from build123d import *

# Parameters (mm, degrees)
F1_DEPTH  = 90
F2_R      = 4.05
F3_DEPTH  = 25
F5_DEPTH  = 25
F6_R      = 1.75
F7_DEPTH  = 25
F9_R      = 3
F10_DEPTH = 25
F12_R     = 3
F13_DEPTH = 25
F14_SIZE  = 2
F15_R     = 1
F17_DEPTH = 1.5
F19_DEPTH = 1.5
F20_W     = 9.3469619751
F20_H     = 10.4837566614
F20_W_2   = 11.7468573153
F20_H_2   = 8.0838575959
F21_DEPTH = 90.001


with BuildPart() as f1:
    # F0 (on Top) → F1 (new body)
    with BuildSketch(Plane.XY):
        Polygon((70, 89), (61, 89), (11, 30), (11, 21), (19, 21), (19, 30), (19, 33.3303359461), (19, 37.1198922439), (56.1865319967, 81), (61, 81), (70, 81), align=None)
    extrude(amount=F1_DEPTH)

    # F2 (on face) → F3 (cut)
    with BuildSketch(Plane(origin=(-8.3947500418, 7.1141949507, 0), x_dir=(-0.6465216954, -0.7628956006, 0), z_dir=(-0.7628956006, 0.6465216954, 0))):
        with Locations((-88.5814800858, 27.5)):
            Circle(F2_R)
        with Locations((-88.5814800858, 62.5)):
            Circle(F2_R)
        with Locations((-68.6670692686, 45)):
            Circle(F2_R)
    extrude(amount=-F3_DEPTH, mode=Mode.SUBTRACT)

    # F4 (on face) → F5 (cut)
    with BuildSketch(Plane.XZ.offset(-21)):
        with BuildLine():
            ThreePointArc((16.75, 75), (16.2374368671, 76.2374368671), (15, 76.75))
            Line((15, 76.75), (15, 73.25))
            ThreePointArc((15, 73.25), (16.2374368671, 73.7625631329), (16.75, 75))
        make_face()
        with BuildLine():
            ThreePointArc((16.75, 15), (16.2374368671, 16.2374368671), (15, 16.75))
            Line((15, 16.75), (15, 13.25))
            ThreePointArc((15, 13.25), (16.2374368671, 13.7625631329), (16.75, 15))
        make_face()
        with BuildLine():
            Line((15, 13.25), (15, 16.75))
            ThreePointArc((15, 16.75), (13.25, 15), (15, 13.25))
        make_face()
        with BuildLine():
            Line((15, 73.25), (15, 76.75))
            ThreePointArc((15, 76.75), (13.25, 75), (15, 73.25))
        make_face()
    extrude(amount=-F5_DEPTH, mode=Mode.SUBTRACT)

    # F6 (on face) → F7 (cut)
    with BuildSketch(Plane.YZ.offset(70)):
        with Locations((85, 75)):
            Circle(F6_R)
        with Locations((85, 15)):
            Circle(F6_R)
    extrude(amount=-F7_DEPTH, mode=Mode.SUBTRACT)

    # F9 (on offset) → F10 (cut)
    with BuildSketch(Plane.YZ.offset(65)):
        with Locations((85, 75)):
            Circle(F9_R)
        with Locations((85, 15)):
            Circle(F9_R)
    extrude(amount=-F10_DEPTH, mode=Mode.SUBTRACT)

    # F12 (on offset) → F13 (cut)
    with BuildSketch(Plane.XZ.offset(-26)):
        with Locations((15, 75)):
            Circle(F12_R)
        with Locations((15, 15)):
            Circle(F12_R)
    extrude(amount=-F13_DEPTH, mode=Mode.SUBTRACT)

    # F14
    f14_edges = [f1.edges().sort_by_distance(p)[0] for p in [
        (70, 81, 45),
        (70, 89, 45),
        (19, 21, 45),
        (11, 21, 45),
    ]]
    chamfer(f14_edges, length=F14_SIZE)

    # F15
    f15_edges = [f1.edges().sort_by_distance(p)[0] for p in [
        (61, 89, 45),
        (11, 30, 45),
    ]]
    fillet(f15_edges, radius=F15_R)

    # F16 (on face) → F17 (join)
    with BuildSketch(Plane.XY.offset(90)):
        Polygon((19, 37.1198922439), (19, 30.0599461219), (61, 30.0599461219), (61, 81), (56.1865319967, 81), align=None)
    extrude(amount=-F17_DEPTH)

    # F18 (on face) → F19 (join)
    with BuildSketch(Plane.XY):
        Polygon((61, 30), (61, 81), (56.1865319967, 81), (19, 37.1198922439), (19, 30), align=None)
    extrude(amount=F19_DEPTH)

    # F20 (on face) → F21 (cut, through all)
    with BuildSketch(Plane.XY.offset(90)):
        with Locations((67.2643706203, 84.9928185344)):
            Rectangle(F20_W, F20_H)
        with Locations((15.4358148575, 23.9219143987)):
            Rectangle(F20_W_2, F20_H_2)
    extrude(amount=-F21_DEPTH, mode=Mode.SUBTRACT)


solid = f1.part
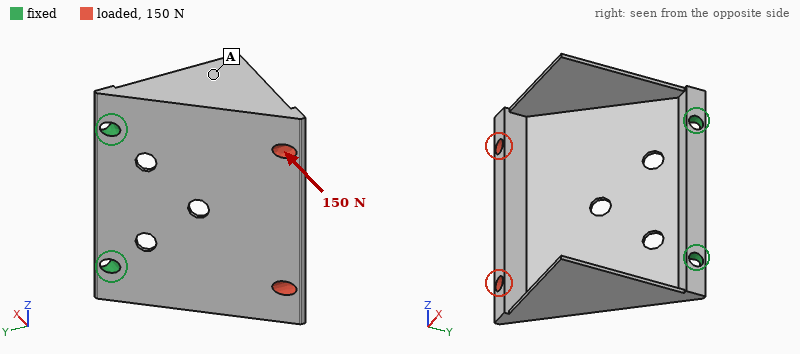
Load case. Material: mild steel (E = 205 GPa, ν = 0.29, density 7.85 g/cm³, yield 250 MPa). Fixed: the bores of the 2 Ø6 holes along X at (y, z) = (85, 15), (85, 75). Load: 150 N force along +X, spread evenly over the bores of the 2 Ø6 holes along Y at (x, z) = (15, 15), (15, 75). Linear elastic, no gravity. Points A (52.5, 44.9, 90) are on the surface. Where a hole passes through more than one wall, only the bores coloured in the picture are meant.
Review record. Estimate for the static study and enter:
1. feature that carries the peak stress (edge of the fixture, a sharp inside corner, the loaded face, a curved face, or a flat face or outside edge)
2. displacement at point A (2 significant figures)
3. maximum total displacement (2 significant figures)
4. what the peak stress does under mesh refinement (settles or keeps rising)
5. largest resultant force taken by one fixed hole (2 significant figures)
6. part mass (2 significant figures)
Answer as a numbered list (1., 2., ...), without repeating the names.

1. a sharp inside corner
2. 0.15 mm
3. 0.30 mm
4. keeps rising
5. 76 N
6. 150 g
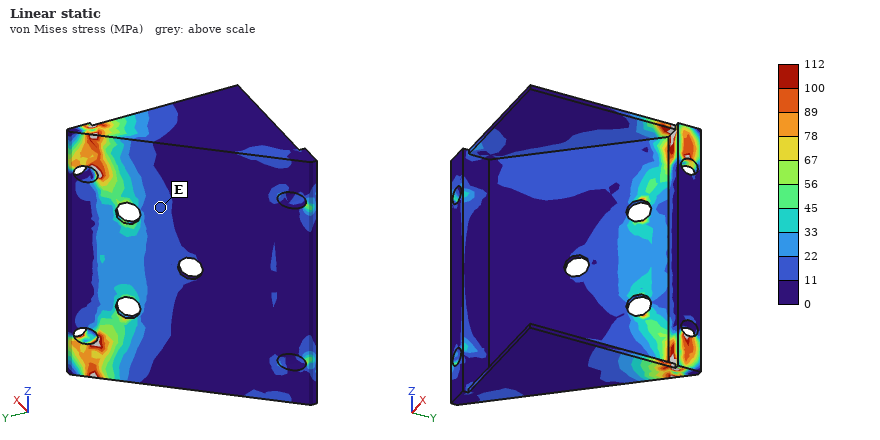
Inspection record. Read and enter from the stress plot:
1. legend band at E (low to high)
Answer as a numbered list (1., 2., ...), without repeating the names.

1. 11 to 22 MPa
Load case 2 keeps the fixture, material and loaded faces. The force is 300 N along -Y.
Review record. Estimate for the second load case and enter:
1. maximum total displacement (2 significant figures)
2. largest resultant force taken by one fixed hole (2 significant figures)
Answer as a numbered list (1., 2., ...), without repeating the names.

1. 0.48 mm
2. 150 N
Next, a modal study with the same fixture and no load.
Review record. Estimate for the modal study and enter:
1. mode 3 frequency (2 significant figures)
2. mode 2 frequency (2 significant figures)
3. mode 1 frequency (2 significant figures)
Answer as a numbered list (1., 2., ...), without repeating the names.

1. 1300 Hz
2. 710 Hz
3. 430 Hz
